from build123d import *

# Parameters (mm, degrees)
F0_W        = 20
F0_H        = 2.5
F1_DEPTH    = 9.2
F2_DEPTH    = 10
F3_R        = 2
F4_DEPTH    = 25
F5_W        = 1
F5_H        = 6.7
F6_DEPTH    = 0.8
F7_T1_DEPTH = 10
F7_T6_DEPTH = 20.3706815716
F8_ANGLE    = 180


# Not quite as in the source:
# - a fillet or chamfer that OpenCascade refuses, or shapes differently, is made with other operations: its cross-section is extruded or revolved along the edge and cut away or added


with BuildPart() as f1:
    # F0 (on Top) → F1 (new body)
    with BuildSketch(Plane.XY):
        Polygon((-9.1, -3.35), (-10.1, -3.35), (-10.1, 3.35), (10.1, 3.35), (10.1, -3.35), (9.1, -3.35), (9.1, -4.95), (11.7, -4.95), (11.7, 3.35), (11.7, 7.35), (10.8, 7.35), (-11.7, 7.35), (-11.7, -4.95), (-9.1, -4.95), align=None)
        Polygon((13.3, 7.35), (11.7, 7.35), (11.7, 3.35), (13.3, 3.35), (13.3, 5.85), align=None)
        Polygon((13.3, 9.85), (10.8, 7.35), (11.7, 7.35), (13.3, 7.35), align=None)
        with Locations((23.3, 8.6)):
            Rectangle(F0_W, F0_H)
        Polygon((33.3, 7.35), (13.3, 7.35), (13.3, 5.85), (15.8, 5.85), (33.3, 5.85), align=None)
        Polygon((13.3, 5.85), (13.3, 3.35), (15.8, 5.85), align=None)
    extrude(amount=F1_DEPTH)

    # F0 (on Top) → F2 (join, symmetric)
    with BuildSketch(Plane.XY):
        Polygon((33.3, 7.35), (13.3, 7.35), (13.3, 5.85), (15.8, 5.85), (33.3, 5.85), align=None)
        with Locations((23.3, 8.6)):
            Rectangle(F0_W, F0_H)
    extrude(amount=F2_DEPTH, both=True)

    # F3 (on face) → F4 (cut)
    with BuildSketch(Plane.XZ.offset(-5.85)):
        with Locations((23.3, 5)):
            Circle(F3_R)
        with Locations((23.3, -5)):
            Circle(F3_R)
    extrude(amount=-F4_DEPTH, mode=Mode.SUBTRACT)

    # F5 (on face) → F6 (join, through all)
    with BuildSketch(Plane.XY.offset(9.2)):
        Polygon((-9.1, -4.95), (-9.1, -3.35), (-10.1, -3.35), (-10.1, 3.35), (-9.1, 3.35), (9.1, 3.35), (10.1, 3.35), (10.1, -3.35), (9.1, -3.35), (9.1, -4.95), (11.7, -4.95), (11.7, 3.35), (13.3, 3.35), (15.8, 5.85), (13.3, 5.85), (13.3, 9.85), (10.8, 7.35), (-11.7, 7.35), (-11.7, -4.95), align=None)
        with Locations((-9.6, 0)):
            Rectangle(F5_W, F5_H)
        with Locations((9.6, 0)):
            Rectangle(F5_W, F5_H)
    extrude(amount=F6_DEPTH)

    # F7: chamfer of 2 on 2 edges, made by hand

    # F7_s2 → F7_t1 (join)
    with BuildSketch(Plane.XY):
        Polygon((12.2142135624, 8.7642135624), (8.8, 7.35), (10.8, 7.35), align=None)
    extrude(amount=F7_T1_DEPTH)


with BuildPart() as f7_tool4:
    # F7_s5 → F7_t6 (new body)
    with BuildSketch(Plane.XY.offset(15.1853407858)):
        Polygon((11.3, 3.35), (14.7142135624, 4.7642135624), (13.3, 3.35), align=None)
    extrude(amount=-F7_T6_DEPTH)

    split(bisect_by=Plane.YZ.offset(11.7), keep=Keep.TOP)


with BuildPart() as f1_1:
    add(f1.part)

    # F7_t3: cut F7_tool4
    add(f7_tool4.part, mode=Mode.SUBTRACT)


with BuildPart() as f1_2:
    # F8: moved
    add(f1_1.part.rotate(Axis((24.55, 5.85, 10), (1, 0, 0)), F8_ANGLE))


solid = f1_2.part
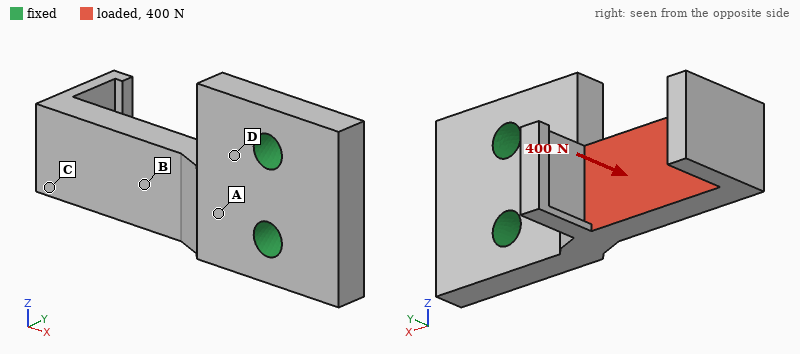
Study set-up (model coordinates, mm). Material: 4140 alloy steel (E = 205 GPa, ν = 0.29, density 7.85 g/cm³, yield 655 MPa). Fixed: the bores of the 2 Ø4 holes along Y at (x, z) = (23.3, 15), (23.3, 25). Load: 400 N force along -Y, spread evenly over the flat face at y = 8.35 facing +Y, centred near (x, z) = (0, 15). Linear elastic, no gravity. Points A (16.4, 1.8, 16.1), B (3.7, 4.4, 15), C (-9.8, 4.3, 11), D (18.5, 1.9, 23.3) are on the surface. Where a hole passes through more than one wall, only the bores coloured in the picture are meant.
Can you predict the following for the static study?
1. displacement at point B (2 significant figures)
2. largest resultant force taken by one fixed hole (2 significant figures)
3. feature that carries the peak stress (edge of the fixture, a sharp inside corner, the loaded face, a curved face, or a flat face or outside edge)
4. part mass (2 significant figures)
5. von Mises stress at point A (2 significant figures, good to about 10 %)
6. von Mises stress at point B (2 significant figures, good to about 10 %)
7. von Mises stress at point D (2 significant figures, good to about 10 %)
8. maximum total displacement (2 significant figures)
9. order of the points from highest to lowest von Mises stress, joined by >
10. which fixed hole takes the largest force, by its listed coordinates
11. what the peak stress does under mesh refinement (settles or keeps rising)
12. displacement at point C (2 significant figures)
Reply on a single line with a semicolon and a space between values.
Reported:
0.073 mm; 330 N; edge of the fixture; 23 g; 180 MPa; 69 MPa; 120 MPa; 0.21 mm; A > D > B > C; (23.3, 15); keeps rising; 0.17 mm
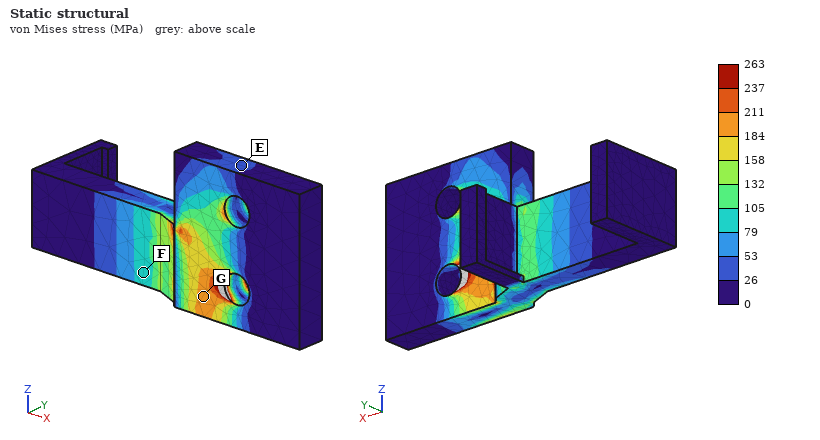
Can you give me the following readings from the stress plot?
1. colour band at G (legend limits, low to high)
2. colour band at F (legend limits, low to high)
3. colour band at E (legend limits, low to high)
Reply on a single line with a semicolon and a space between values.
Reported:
184 to 211 MPa; 79 to 105 MPa; 26 to 53 MPa
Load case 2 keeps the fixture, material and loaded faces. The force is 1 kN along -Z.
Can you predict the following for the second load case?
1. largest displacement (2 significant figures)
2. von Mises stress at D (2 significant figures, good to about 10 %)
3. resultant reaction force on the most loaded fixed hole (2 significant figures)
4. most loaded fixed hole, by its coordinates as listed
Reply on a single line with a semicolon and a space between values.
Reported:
97 µm; 88 MPa; 2.1 kN; (23.3, 25)
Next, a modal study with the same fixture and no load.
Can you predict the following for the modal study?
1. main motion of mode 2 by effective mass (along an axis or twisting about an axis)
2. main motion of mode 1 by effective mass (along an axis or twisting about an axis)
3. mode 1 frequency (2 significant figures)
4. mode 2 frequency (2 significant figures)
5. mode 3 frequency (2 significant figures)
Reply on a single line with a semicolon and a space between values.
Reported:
along Z; along Y; 2700 Hz; 6600 Hz; 11 kHz
